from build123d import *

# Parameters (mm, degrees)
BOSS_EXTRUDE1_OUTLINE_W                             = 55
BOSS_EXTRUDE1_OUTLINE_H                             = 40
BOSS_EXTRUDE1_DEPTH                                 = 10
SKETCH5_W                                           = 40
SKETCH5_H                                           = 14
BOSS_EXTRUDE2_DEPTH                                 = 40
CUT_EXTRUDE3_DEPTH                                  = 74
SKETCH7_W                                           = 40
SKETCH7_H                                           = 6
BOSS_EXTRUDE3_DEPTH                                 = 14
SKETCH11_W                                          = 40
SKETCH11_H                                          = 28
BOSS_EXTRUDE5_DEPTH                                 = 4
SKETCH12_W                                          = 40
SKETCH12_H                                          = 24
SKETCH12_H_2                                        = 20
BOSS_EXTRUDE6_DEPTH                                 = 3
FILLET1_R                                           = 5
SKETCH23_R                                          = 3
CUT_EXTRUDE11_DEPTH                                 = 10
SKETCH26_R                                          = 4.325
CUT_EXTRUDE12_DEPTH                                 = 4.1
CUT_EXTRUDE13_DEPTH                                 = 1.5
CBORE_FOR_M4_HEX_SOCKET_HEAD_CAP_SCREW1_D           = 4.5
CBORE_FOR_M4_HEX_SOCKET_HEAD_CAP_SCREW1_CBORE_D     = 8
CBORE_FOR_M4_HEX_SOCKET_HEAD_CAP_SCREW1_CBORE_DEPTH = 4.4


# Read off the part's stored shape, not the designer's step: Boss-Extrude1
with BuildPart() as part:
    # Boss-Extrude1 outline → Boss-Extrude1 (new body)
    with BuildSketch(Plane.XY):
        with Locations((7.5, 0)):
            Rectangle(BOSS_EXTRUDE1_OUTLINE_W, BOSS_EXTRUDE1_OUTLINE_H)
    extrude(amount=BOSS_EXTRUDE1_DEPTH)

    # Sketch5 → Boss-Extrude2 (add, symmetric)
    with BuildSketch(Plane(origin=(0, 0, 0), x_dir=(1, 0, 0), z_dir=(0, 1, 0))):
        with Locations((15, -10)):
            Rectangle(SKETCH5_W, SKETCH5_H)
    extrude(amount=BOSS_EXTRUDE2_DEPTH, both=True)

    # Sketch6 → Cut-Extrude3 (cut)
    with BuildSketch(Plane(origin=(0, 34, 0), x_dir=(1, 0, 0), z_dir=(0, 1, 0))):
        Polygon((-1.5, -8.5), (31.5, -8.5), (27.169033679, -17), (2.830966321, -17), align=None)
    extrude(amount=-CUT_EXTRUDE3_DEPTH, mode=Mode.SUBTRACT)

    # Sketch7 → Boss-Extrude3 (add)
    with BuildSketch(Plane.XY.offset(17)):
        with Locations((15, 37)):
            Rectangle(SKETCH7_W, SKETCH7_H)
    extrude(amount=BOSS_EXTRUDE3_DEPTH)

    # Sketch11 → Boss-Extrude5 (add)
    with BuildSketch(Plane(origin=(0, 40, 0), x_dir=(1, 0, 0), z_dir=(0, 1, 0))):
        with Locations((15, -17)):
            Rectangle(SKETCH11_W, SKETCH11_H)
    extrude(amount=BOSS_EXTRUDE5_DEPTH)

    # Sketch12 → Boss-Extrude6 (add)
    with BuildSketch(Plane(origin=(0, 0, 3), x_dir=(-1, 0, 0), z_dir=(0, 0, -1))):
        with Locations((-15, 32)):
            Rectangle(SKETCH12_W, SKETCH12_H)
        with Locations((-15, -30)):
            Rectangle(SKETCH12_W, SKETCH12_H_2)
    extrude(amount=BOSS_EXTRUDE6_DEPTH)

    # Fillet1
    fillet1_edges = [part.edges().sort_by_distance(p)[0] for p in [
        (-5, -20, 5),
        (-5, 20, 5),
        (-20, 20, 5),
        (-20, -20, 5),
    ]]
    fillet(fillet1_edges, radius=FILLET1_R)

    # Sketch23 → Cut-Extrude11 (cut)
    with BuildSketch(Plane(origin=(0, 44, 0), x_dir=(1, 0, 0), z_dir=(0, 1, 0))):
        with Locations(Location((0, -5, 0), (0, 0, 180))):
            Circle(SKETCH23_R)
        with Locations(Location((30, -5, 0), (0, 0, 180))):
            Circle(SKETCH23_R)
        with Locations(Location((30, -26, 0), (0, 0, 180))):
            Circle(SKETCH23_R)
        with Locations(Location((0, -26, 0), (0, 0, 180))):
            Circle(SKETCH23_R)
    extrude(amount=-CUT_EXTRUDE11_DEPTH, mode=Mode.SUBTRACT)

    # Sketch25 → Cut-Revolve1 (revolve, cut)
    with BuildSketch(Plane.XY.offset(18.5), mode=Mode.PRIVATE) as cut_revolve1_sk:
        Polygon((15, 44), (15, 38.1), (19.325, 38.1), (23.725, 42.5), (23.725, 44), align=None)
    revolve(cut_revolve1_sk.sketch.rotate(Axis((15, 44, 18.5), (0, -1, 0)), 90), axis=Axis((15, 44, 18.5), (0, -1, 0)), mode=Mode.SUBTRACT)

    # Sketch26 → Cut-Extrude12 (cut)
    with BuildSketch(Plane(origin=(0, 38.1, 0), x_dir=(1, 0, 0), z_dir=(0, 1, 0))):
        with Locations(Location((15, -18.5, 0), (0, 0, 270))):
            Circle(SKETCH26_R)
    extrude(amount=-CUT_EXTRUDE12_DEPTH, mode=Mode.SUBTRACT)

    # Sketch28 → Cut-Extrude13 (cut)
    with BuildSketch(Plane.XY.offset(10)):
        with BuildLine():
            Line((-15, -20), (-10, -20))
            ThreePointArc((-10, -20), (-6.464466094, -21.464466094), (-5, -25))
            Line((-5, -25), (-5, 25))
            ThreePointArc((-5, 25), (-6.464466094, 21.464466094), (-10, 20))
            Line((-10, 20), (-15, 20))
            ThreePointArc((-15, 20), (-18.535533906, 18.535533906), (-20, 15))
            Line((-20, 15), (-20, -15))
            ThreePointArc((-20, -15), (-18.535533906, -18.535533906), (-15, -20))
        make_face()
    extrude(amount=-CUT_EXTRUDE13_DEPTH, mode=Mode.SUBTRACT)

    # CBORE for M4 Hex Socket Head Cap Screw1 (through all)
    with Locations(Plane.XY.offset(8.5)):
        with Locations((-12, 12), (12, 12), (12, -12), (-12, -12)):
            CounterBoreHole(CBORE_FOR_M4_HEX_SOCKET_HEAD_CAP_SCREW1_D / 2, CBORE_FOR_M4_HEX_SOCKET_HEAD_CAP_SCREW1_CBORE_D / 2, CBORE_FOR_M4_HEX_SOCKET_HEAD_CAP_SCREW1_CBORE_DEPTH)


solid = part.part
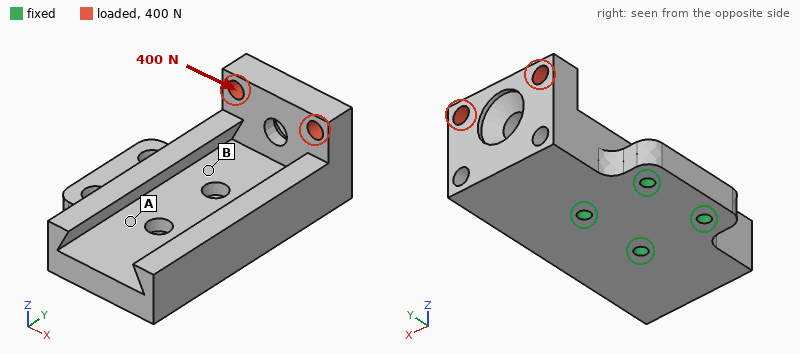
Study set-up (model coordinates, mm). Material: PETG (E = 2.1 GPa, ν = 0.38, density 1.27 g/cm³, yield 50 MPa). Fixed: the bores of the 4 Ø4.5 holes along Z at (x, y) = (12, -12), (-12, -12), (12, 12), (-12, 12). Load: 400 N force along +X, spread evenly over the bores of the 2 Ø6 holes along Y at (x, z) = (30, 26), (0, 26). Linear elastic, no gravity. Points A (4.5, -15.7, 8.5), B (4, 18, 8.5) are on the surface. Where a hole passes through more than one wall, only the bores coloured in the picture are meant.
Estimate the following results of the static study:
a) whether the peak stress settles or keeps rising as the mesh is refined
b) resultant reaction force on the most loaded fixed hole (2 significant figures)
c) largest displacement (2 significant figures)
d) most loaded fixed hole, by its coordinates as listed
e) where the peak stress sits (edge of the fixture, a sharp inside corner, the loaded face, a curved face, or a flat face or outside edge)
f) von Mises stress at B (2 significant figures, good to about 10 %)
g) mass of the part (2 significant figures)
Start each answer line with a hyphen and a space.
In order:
- keeps rising
- 570 N
- 0.99 mm
- (-12, 12)
- edge of the fixture
- 10 MPa
- 59 g
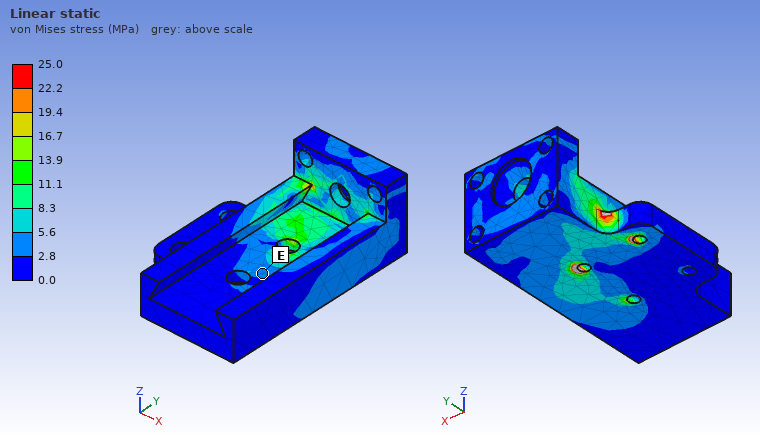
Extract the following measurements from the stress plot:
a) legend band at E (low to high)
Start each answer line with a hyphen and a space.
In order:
- 2.8 to 5.6 MPa
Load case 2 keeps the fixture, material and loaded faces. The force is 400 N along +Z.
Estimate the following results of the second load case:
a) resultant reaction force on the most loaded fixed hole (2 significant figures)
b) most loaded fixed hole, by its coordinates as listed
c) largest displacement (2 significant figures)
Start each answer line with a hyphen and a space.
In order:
- 690 N
- (12, 12)
- 1.0 mm
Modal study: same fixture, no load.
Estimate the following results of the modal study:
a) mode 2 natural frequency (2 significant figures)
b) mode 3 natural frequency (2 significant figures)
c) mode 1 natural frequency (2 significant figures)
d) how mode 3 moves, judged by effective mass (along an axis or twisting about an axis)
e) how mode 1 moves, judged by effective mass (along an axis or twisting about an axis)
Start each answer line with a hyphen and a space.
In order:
- 1300 Hz
- 1600 Hz
- 900 Hz
- along Z
- along Z
